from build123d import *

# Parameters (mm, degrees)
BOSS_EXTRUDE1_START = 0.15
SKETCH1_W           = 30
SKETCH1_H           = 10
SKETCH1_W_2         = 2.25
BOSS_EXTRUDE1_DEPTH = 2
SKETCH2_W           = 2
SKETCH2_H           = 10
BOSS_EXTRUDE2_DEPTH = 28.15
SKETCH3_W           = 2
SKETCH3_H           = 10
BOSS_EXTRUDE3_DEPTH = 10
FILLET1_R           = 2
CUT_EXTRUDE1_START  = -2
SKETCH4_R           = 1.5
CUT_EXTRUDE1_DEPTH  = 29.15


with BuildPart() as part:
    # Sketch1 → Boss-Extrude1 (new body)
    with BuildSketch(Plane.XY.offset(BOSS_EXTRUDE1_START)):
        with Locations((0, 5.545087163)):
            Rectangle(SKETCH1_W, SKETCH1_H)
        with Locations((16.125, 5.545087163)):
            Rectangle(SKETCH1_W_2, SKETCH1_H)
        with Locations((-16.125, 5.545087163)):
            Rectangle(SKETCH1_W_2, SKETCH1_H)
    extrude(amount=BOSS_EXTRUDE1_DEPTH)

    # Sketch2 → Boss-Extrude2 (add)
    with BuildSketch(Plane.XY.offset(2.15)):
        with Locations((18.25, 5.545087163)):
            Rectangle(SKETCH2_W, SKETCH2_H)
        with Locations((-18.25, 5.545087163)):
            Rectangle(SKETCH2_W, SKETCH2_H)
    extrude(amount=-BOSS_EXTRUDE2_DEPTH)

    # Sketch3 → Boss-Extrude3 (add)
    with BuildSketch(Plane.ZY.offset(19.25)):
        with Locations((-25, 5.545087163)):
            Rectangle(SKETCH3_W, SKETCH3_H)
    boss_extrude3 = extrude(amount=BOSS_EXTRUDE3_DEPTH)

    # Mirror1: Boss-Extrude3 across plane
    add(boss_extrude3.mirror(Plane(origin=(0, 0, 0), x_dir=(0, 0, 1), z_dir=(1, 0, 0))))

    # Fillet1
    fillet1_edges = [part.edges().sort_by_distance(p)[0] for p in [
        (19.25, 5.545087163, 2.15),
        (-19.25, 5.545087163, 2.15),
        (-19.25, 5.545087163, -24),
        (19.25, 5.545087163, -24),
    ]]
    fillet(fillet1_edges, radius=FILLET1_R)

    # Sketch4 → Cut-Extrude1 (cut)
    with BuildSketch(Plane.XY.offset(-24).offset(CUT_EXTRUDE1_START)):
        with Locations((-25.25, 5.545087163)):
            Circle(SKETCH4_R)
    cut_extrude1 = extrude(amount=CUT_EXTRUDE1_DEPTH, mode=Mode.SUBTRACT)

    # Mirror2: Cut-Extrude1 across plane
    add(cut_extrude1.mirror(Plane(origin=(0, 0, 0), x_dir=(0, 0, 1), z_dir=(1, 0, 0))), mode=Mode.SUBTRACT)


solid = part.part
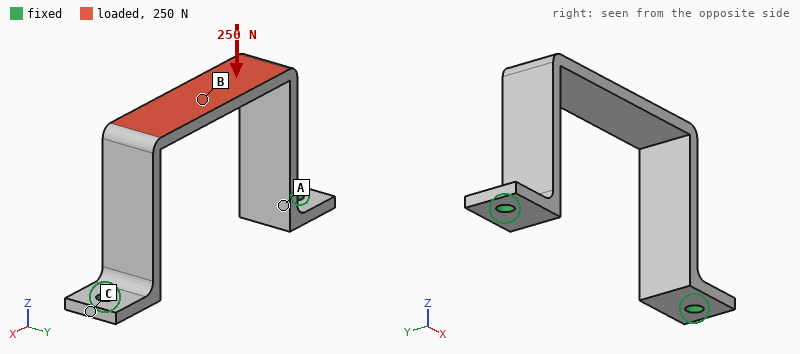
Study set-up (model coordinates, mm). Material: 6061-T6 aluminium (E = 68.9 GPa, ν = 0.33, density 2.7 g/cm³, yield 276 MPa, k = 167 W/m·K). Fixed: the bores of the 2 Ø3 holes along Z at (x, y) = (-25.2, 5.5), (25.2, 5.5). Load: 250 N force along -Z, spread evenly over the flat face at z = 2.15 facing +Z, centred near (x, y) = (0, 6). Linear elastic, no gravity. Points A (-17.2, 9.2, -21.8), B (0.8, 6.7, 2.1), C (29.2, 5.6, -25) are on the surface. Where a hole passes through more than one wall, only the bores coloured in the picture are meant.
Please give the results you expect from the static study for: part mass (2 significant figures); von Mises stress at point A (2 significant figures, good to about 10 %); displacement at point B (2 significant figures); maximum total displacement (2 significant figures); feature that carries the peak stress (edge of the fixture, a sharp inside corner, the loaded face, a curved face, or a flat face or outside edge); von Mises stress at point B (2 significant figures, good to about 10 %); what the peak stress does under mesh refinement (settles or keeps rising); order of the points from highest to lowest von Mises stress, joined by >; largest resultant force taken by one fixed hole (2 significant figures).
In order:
5.9 g
33 MPa
0.14 mm
0.15 mm
edge of the fixture
85 MPa
keeps rising
B > A > C
130 N
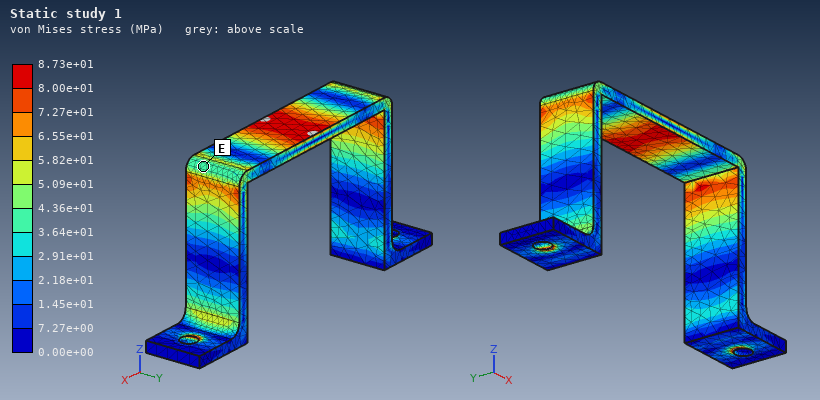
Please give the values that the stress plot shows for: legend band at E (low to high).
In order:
3.64e+01 to 4.36e+01 MPa
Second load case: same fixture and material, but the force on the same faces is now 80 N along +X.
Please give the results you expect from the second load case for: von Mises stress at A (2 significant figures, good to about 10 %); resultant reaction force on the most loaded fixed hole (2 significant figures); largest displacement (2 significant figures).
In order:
57 MPa
50 N
0.24 mm
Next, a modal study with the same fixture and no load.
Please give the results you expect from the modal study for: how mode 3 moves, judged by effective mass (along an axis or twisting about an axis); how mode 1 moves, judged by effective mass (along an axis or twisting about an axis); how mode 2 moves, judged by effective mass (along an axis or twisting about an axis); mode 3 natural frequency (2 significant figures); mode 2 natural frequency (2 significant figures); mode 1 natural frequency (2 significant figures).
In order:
twisting about Z
along X
along Y
3200 Hz
1900 Hz
1700 Hz
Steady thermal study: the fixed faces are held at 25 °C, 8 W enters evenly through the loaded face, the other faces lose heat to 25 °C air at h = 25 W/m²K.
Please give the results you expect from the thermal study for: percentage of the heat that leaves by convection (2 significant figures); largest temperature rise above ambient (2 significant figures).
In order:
14 %
43 K
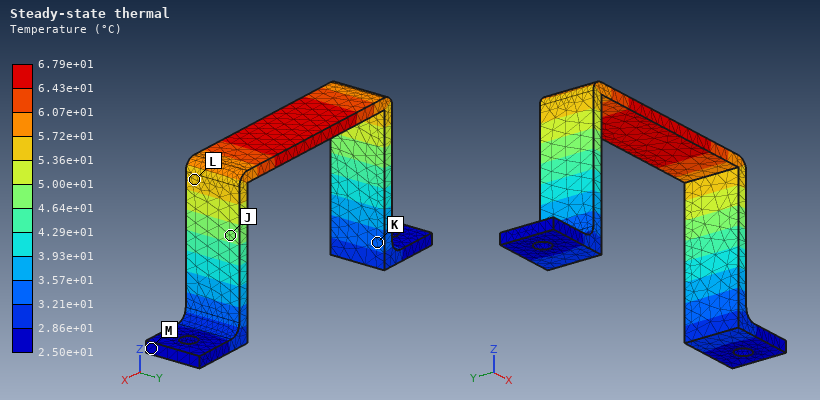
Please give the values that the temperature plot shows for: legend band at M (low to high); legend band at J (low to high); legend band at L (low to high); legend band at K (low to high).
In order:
2.50e+01 to 2.86e+01 °C
4.64e+01 to 5.00e+01 °C
5.36e+01 to 5.72e+01 °C
3.21e+01 to 3.57e+01 °C
